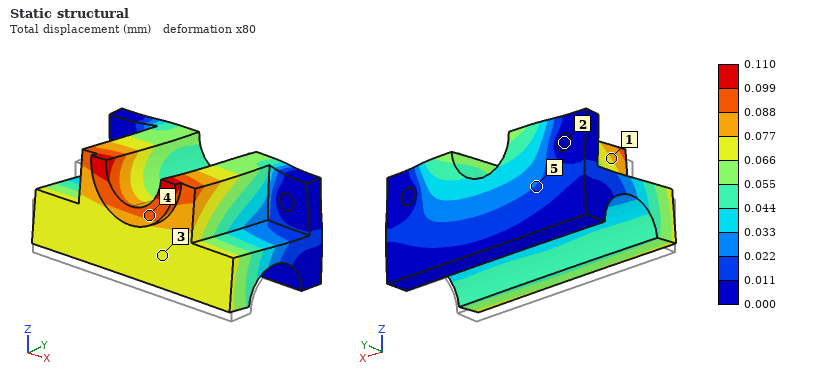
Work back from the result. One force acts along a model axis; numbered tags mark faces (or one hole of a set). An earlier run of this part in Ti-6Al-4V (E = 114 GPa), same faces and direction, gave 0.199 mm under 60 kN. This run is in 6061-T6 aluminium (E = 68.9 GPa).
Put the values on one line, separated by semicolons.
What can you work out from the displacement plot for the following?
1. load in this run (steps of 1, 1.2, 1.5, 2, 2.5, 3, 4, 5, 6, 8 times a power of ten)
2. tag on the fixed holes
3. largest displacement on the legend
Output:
20 kN; 2; 0.110 mm
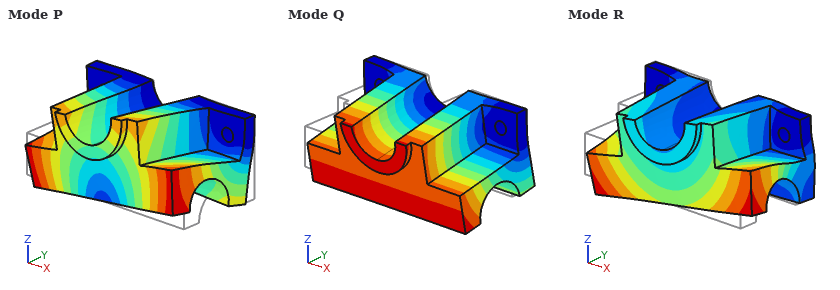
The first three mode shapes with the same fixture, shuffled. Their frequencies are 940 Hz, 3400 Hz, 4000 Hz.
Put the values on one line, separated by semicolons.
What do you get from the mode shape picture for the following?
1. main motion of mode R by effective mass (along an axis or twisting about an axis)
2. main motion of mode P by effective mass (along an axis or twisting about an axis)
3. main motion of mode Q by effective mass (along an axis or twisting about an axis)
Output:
along X; along X; along Z
